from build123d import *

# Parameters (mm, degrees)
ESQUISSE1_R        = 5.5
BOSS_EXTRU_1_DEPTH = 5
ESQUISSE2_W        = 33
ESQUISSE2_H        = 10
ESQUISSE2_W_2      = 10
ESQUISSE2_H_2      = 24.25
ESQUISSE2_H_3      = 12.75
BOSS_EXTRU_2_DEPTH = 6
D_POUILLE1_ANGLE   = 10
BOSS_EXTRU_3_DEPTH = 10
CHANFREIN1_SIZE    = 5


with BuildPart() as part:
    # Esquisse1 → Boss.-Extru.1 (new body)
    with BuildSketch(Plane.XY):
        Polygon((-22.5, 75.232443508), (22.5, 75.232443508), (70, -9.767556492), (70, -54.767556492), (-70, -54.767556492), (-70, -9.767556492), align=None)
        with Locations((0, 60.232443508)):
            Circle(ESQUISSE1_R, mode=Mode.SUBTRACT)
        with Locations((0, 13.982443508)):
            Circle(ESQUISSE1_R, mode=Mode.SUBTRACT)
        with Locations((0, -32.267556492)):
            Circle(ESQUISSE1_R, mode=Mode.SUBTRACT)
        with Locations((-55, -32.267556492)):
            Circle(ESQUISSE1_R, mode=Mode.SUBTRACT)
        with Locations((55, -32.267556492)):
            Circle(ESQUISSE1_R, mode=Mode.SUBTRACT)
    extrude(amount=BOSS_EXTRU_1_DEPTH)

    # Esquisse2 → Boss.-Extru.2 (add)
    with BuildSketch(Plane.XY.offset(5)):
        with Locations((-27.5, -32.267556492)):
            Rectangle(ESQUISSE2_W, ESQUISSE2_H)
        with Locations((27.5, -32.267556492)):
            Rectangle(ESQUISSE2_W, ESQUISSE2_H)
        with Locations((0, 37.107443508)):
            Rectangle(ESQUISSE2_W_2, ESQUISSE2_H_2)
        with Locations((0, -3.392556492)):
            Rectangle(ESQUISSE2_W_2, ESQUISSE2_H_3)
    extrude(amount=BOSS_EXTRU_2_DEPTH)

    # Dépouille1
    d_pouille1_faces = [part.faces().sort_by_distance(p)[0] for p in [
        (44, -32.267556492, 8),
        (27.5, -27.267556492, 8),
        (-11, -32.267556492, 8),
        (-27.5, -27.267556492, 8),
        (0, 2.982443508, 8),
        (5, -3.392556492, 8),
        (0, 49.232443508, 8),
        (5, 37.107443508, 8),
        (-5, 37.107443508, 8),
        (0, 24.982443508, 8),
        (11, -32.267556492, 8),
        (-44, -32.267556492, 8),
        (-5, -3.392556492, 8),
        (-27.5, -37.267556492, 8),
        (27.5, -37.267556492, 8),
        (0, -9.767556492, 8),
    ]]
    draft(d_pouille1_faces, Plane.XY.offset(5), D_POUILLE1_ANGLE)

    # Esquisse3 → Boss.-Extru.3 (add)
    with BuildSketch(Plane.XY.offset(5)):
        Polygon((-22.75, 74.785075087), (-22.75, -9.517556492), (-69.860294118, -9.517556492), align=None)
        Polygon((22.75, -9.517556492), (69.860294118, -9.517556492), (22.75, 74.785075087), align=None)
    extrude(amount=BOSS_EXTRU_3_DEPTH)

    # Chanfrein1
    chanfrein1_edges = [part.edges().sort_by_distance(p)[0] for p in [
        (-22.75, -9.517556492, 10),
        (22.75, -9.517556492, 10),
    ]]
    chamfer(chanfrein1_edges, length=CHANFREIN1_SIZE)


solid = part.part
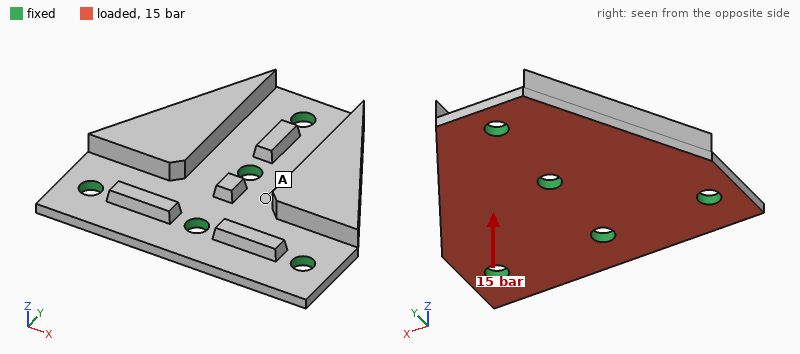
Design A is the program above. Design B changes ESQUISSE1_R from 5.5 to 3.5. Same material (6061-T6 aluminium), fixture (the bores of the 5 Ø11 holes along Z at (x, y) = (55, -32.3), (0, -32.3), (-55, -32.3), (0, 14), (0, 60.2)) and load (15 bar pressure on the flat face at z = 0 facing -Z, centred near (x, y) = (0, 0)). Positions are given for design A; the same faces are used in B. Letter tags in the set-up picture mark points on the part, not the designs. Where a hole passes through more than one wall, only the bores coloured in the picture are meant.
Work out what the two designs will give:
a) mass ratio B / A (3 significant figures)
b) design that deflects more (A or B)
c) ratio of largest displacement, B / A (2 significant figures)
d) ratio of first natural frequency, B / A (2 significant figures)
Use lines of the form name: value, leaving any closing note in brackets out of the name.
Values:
mass ratio B / A: 1.01
design that deflects more: B
ratio of largest displacement, B / A: 1.2
ratio of first natural frequency, B / A: 0.86
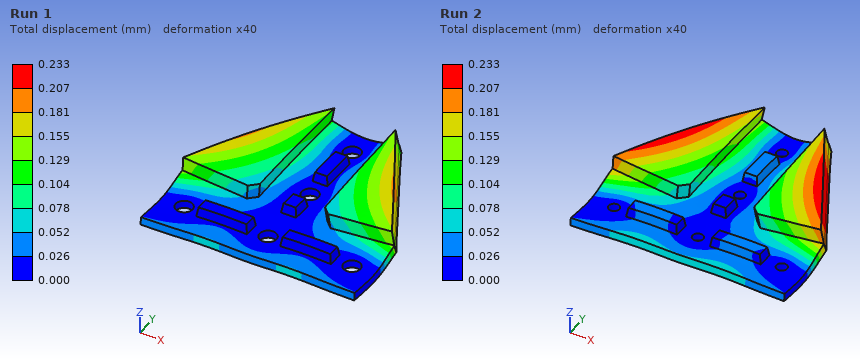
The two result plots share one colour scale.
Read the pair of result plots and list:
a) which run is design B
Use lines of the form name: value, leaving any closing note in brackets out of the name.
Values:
which run is design B: Run 2
